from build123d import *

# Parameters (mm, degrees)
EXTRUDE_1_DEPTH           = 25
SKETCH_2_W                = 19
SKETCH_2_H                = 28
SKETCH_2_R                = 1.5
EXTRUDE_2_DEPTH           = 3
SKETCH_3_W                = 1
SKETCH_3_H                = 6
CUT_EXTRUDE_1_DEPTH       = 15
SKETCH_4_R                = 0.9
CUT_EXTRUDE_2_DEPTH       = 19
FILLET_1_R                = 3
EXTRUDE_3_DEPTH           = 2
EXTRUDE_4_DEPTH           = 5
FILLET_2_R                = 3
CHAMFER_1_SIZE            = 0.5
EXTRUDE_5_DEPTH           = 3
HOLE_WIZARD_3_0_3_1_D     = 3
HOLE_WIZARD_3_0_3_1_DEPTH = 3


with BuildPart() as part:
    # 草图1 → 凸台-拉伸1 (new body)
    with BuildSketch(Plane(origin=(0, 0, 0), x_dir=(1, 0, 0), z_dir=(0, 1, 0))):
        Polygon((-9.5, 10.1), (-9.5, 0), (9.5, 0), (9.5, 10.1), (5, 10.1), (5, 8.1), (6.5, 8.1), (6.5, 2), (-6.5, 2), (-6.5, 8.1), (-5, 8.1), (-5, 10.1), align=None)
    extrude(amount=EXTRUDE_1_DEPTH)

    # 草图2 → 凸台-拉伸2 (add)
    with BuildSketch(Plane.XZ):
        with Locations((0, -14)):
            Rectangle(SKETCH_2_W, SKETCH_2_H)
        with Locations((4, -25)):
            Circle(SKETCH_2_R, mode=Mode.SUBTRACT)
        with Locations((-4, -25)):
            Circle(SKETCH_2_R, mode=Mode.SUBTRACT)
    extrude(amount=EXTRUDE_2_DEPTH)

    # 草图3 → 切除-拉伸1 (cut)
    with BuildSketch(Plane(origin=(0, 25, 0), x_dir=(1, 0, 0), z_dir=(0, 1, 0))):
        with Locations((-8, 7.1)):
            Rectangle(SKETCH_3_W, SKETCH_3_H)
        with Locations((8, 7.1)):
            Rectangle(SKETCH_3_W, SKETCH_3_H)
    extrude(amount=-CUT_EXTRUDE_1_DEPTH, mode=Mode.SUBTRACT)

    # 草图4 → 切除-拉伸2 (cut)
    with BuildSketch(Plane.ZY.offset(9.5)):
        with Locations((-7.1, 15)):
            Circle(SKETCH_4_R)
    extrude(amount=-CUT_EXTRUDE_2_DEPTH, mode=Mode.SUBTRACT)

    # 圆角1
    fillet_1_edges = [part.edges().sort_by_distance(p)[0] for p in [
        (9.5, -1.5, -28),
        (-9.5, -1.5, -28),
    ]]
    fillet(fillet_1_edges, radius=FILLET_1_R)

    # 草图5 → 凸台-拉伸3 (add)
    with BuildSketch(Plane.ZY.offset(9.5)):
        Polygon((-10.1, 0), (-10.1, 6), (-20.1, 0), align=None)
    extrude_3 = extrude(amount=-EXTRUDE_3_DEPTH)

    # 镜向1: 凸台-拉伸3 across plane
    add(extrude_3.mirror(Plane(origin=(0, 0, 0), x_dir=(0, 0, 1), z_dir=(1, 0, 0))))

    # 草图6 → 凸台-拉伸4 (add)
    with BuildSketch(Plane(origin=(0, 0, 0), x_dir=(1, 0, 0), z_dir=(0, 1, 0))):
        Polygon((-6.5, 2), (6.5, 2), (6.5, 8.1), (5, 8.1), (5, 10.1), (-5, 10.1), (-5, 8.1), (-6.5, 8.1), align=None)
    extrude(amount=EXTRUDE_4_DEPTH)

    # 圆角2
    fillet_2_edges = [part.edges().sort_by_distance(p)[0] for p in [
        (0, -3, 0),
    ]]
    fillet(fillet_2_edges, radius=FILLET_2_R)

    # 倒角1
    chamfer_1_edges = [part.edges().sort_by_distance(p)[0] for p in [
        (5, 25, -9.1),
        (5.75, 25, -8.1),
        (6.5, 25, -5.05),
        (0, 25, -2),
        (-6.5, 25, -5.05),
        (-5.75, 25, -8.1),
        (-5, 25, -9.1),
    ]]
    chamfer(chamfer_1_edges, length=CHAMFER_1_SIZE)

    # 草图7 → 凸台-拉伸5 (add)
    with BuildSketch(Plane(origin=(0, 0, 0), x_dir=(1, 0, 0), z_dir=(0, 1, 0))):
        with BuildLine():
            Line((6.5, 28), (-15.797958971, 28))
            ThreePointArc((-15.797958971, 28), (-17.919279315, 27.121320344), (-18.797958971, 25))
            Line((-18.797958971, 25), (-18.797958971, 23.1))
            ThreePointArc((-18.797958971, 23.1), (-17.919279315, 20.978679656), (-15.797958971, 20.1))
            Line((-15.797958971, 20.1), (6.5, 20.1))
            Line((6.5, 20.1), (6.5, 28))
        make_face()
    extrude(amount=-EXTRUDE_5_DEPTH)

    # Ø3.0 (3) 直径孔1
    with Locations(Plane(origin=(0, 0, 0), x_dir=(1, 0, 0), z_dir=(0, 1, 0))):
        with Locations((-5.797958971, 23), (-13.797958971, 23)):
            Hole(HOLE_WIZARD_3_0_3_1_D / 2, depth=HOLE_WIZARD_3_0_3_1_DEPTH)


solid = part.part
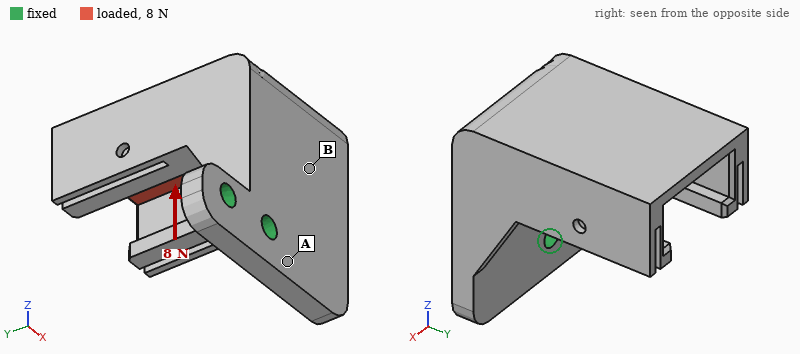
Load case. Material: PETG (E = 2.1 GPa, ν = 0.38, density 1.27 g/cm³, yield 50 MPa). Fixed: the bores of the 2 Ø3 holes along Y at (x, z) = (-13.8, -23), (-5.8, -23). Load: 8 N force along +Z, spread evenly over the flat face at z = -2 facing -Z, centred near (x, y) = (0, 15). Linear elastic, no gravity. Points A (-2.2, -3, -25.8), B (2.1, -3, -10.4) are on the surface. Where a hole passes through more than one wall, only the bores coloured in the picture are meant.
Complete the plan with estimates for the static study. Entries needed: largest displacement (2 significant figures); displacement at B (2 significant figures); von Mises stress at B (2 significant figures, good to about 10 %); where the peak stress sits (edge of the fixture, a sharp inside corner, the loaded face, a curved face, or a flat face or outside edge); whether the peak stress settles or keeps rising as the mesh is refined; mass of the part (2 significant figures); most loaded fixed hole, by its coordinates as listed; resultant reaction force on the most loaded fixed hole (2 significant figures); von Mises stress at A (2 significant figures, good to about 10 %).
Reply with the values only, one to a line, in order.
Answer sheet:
0.50 mm
0.12 mm
1.2 MPa
edge of the fixture
keeps rising
5.7 g
(-5.8, -23)
11 N
2.8 MPa
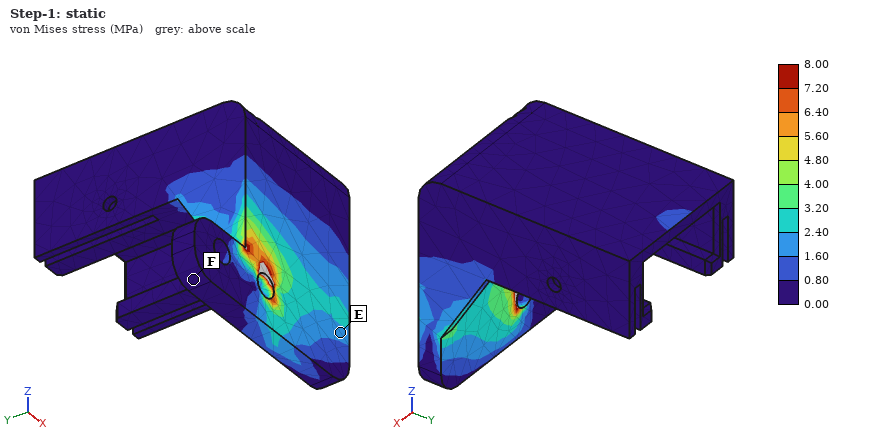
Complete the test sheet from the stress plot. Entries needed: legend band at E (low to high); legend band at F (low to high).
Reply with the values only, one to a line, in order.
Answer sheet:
1.60 to 2.40 MPa
0.00 to 0.80 MPa
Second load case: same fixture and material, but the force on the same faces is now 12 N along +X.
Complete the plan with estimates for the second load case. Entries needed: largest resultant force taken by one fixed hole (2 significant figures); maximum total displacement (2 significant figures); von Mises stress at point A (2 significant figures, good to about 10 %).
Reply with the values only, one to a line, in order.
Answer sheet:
21 N
0.55 mm
6.3 MPa
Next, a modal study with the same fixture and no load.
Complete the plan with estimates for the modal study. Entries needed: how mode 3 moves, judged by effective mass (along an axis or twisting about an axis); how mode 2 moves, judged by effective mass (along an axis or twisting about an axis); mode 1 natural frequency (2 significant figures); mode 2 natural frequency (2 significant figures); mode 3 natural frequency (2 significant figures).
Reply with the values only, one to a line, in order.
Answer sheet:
along X
along X
370 Hz
560 Hz
1400 Hz
